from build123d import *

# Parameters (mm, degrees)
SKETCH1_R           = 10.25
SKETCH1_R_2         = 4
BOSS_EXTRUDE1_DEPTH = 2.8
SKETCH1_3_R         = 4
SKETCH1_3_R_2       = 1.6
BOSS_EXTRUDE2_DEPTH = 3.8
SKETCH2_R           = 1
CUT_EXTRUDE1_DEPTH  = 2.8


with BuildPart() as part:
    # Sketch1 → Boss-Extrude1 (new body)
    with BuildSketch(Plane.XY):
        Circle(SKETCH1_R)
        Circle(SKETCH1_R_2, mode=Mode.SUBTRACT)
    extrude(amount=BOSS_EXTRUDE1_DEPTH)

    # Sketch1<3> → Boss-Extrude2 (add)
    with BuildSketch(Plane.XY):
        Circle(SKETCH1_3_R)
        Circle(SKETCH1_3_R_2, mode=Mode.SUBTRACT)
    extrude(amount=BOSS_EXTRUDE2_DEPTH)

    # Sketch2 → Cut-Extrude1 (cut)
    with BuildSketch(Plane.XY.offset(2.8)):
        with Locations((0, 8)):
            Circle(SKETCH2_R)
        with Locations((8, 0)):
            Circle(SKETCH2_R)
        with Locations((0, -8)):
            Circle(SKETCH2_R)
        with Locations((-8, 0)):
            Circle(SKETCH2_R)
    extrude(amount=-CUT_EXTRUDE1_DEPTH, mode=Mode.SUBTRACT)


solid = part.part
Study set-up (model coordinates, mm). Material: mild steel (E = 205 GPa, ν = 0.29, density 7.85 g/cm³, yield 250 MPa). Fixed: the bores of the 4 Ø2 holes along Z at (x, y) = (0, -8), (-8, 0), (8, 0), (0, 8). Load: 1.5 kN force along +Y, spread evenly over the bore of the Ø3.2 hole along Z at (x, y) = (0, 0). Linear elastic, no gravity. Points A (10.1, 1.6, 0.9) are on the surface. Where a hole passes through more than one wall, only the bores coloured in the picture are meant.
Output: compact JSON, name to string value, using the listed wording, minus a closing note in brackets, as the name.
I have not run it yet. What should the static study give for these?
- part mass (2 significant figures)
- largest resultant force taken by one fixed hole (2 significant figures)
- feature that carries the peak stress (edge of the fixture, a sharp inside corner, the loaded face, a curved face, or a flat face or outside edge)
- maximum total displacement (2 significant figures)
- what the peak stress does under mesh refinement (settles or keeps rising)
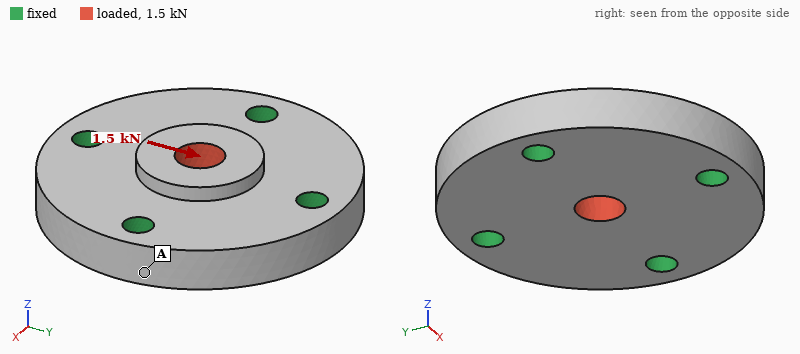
{"part mass": "7.1 g", "largest resultant force taken by one fixed hole": "500 N", "feature that carries the peak stress": "edge of the fixture", "maximum total displacement": "1.5 µm", "what the peak stress does under mesh refinement": "keeps rising"}
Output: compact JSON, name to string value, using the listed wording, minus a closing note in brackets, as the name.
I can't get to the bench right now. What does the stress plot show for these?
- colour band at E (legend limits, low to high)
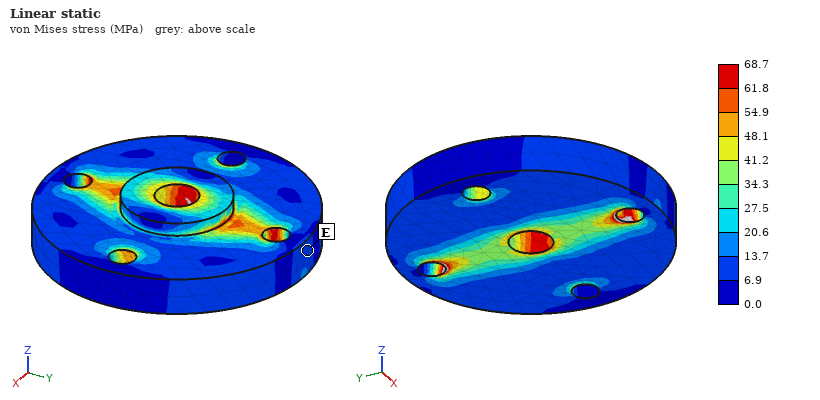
{"colour band at E": "6.9 to 13.7 MPa"}
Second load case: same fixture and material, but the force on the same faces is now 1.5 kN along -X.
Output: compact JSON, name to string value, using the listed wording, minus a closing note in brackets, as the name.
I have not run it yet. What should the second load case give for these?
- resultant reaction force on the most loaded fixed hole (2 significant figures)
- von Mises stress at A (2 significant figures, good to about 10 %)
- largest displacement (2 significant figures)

{"resultant reaction force on the most loaded fixed hole": "500 N", "von Mises stress at A": "6.9 MPa", "largest displacement": "1.5 µm"}
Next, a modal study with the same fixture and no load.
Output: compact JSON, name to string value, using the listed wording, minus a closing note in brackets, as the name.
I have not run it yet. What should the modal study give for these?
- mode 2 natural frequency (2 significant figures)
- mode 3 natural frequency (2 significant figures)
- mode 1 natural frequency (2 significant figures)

{"mode 2 natural frequency": "74 kHz", "mode 3 natural frequency": "76 kHz", "mode 1 natural frequency": "73 kHz"}
